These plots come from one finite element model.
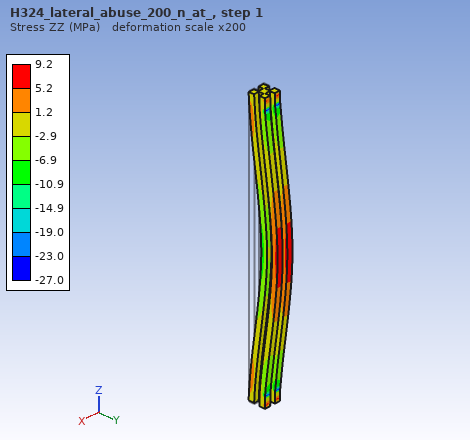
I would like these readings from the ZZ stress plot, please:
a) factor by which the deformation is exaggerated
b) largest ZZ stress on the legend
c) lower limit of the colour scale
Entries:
200
9.2 MPa
-27.0 MPa
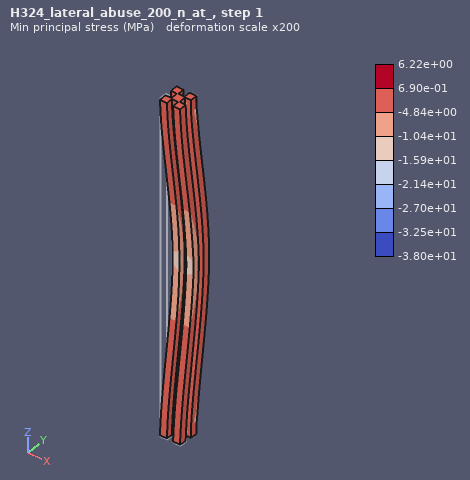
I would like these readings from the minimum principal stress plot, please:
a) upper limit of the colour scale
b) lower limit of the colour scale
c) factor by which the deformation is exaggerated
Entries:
6.22e+00 MPa
-3.80e+01 MPa
200
